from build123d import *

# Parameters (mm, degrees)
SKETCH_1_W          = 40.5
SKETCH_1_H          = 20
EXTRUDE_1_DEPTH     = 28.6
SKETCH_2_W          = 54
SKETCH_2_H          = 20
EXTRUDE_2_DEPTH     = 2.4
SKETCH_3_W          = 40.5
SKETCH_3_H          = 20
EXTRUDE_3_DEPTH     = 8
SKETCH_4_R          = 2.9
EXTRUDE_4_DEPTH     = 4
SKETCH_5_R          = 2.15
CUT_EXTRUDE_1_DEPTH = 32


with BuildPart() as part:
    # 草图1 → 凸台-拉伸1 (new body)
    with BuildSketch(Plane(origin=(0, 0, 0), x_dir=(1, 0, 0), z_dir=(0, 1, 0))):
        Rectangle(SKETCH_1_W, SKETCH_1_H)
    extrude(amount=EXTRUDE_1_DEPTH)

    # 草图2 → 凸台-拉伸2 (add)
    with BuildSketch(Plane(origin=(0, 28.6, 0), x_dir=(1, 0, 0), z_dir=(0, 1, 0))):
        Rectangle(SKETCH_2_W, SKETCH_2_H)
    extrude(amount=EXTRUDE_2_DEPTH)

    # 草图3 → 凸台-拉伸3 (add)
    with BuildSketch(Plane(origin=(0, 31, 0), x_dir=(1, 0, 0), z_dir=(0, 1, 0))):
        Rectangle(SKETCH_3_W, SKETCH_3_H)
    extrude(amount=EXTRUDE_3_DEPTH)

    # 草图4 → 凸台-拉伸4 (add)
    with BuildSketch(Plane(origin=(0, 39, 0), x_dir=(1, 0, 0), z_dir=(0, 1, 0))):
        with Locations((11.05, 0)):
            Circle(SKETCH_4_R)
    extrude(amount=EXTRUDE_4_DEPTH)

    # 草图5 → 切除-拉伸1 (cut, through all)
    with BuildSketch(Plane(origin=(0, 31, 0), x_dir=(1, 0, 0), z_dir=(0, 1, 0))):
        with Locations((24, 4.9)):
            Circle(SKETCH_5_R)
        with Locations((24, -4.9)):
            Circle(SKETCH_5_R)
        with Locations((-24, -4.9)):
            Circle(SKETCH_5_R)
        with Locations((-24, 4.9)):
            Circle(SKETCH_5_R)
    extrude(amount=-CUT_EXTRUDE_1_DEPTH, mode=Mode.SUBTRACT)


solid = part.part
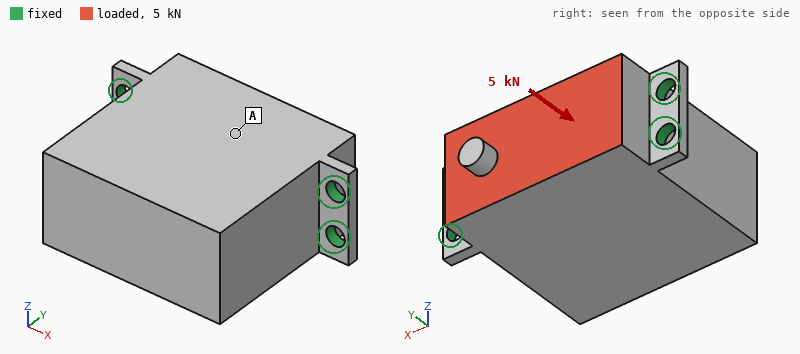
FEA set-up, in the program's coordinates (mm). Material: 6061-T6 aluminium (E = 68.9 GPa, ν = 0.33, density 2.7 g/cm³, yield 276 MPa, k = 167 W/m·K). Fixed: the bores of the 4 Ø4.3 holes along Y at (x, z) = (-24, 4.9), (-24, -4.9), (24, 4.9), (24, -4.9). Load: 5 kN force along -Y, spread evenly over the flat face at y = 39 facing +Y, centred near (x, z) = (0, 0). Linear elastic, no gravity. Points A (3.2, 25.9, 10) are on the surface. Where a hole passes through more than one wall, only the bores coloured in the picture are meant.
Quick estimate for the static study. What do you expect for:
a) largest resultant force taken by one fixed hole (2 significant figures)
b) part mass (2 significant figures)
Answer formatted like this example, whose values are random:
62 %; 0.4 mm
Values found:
1.3 kN; 87 g
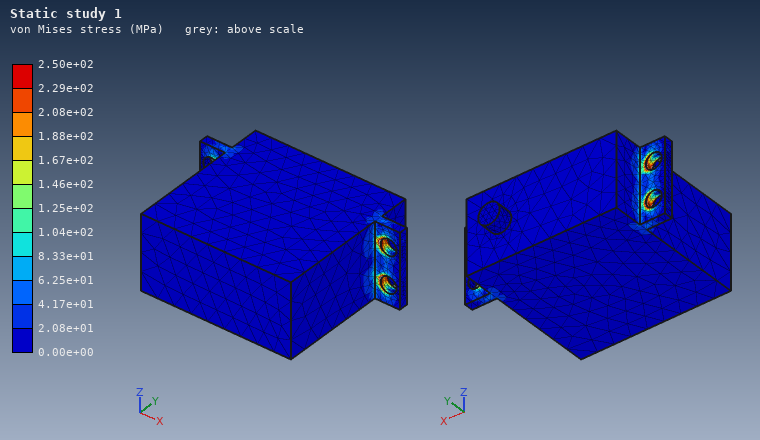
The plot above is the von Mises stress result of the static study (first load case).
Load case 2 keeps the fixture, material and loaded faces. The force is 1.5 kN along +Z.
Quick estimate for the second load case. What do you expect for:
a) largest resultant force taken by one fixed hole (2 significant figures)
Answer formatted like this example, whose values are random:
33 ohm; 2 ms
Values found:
710 N
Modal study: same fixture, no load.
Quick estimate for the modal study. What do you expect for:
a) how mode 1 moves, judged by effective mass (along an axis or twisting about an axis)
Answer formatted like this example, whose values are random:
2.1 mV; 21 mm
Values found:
along Z
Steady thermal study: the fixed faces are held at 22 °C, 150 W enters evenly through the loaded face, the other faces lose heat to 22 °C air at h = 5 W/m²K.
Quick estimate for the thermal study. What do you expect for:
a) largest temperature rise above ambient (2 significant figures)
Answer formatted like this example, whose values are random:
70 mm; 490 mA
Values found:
55 K
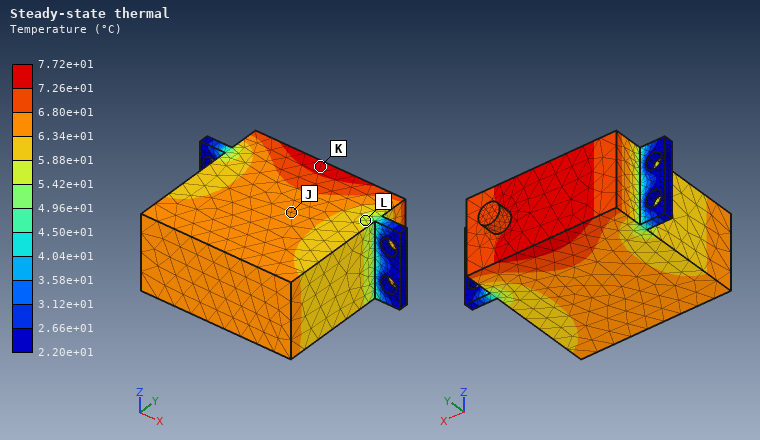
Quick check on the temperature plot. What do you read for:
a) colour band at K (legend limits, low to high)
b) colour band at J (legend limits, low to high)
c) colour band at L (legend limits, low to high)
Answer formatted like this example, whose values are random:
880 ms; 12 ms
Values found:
7.26e+01 to 7.72e+01 °C; 6.34e+01 to 6.80e+01 °C; 5.42e+01 to 5.88e+01 °C
